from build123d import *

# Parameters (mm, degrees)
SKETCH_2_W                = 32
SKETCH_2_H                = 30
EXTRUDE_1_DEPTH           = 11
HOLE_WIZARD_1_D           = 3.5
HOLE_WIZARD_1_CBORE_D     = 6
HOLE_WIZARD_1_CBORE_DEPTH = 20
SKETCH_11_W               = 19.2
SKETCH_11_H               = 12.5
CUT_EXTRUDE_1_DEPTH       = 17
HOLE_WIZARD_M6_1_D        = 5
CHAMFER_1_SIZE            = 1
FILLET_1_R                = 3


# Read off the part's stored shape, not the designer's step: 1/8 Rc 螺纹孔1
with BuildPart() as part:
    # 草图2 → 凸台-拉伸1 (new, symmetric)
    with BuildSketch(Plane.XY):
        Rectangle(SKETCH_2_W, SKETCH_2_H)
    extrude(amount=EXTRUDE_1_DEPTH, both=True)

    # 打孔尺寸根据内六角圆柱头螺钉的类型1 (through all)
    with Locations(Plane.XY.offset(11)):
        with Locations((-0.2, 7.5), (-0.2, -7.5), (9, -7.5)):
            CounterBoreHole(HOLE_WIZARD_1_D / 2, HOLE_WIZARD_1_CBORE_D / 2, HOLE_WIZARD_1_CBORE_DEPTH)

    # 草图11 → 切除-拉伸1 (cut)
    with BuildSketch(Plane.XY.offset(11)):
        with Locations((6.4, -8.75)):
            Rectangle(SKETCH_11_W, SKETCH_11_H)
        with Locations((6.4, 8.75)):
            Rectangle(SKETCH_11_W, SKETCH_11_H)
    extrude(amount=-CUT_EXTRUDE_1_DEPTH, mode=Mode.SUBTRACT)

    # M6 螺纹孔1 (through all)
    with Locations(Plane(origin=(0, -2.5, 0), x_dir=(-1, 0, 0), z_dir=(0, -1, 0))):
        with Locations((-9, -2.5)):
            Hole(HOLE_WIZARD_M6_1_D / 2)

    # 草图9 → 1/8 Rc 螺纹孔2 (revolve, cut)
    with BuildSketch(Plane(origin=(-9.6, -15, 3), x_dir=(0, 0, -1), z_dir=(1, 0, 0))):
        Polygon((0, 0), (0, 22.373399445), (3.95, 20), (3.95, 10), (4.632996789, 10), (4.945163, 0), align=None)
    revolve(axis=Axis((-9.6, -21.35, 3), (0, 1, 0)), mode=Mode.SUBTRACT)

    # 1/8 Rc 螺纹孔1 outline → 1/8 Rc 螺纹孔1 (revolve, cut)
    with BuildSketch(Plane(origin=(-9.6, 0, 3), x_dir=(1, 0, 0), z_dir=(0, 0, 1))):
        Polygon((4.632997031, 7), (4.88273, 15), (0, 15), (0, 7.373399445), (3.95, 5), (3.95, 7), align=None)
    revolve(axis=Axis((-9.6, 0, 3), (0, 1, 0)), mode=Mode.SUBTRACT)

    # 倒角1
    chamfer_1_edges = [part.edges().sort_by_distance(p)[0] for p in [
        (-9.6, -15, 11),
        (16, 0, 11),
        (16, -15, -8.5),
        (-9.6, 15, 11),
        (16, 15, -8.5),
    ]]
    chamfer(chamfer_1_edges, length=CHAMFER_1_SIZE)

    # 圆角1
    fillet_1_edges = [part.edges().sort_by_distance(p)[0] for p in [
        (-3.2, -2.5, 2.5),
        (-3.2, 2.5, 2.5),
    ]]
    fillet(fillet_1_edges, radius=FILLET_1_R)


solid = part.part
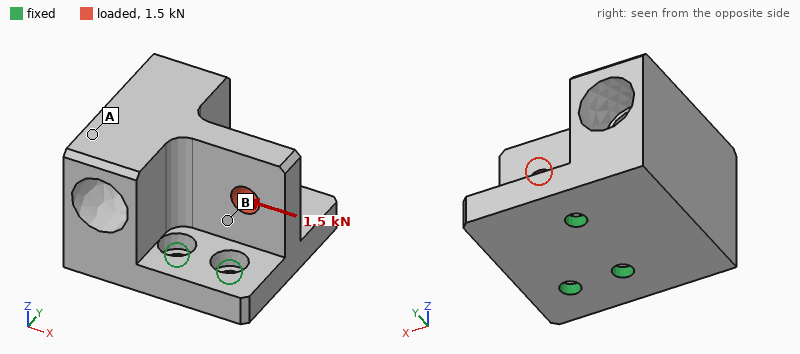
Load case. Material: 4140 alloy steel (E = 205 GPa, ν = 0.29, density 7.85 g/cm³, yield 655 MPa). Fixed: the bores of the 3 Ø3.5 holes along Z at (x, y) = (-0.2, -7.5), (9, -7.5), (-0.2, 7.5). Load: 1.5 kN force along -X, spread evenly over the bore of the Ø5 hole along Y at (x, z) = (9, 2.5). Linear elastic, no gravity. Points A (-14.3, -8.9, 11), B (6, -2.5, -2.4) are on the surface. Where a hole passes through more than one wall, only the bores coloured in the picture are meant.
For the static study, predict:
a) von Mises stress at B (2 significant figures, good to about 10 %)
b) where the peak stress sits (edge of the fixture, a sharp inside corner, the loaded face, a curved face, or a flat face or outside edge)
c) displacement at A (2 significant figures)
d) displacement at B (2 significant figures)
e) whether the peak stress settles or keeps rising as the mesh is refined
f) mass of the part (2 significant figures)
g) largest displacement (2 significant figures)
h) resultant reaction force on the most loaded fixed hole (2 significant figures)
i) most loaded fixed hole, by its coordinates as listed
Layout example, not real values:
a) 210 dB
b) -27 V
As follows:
a) 55 MPa
b) edge of the fixture
c) 24 µm
d) 8.8 µm
e) keeps rising
f) 84 g
g) 25 µm
h) 1.6 kN
i) (9, -7.5)
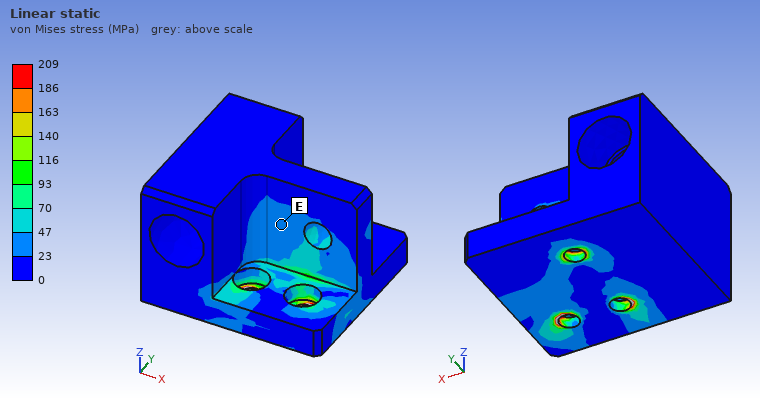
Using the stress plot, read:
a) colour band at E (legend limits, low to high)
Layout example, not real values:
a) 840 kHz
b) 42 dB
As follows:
a) 23 to 47 MPa
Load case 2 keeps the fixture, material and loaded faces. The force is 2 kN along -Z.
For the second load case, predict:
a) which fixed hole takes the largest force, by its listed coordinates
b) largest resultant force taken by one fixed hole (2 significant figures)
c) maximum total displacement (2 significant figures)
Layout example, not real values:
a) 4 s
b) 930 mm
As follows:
a) (9, -7.5)
b) 1.6 kN
c) 20 µm
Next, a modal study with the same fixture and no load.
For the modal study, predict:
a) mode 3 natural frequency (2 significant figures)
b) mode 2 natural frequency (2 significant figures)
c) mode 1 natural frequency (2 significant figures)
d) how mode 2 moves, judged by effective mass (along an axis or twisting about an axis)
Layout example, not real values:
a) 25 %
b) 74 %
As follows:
a) 16 kHz
b) 9600 Hz
c) 5400 Hz
d) along Y
